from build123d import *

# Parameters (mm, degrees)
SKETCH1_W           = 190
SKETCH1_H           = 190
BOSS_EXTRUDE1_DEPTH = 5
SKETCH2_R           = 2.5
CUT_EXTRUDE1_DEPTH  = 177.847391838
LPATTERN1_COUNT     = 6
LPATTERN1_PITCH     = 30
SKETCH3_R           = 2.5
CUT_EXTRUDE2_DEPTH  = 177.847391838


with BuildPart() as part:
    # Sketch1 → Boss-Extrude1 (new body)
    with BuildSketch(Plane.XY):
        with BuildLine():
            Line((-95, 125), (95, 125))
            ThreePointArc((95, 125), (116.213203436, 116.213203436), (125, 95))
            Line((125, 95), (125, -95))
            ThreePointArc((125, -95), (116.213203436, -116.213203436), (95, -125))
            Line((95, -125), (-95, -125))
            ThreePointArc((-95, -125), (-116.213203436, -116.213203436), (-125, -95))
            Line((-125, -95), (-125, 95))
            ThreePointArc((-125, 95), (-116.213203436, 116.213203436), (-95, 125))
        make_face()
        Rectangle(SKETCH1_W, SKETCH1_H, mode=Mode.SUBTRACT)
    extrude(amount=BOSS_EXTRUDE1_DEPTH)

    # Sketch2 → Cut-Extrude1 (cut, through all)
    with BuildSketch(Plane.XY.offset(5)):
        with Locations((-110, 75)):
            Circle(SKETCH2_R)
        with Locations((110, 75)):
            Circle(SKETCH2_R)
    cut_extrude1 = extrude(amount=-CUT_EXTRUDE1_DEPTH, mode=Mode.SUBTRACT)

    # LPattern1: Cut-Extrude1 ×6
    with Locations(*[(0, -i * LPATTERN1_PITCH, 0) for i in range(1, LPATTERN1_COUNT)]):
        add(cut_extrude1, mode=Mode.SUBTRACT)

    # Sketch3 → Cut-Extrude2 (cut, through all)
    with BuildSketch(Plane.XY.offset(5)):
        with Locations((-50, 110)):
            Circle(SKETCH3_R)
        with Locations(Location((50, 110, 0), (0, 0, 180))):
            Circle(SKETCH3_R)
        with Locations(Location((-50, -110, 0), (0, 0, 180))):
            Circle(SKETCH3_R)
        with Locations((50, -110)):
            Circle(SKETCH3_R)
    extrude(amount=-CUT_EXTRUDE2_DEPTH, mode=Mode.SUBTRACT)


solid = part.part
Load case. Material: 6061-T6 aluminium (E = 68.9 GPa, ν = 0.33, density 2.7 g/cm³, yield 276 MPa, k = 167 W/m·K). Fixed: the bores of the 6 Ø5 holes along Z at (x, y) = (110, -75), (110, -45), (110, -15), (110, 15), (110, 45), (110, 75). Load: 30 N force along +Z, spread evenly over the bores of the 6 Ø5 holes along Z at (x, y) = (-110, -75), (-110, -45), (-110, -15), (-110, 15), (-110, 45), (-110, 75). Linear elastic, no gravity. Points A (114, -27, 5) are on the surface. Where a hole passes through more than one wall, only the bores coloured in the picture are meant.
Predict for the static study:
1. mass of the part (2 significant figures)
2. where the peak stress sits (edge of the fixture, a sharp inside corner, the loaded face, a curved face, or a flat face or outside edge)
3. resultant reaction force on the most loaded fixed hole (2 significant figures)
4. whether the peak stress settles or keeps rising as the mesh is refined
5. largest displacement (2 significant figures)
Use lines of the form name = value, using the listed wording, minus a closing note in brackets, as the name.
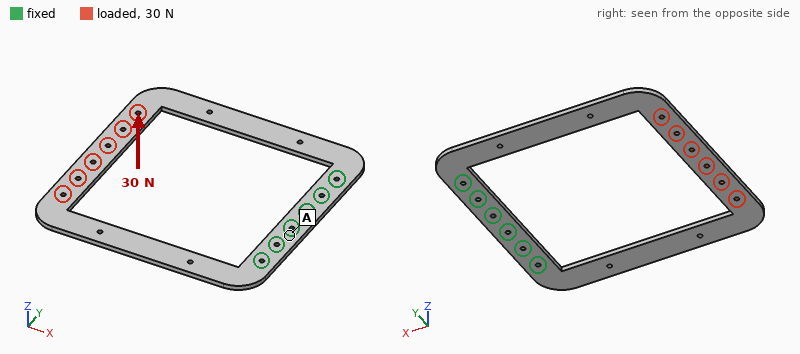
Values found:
mass of the part = 340 g
where the peak stress sits = edge of the fixture
resultant reaction force on the most loaded fixed hole = 19 N
whether the peak stress settles or keeps rising as the mesh is refined = keeps rising
largest displacement = 3.4 mm
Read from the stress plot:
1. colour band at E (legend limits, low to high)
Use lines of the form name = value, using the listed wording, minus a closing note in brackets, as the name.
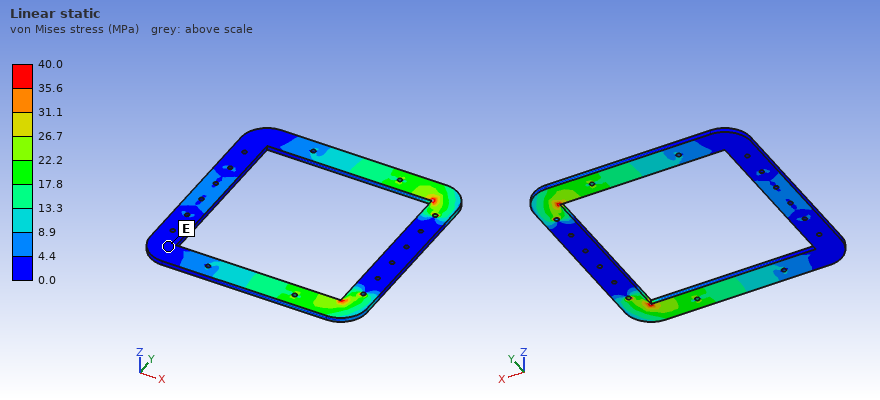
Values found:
colour band at E = 0.0 to 4.4 MPa
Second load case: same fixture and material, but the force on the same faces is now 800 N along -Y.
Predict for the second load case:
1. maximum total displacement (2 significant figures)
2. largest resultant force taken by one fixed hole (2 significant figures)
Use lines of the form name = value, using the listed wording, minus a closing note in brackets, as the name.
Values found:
maximum total displacement = 1.1 mm
largest resultant force taken by one fixed hole = 1.8 kN
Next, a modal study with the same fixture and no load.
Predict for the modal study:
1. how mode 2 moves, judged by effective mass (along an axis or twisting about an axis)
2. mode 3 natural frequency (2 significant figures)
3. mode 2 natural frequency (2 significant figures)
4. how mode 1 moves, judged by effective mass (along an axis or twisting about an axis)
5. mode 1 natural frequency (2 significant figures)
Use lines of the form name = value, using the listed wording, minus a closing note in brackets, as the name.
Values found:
how mode 2 moves, judged by effective mass = twisting about X
mode 3 natural frequency = 300 Hz
mode 2 natural frequency = 100 Hz
how mode 1 moves, judged by effective mass = along Z
mode 1 natural frequency = 44 Hz
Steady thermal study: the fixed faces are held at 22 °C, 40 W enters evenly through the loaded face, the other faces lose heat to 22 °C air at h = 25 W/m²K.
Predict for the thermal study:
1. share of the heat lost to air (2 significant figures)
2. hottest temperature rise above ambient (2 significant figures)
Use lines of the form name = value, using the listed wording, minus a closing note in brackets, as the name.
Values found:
share of the heat lost to air = 88 %
hottest temperature rise above ambient = 68 K
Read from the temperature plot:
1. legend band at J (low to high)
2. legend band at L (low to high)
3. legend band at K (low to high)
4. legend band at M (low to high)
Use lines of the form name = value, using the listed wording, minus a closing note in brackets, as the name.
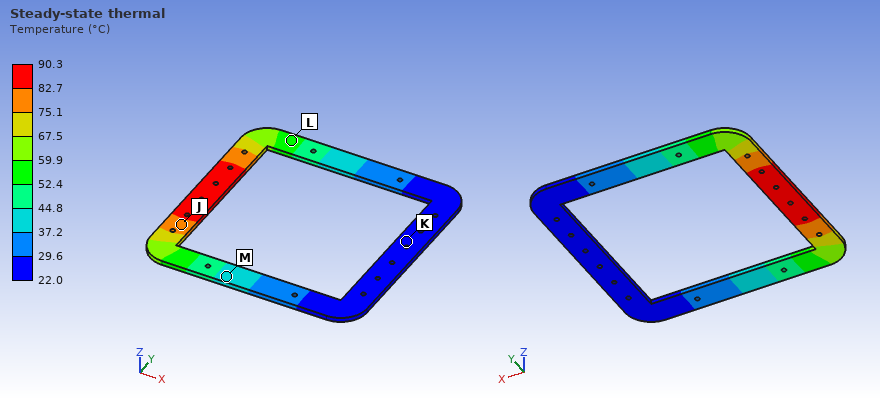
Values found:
legend band at J = 75.1 to 82.7 °C
legend band at L = 52.4 to 59.9 °C
legend band at K = 22.0 to 29.6 °C
legend band at M = 37.2 to 44.8 °C
